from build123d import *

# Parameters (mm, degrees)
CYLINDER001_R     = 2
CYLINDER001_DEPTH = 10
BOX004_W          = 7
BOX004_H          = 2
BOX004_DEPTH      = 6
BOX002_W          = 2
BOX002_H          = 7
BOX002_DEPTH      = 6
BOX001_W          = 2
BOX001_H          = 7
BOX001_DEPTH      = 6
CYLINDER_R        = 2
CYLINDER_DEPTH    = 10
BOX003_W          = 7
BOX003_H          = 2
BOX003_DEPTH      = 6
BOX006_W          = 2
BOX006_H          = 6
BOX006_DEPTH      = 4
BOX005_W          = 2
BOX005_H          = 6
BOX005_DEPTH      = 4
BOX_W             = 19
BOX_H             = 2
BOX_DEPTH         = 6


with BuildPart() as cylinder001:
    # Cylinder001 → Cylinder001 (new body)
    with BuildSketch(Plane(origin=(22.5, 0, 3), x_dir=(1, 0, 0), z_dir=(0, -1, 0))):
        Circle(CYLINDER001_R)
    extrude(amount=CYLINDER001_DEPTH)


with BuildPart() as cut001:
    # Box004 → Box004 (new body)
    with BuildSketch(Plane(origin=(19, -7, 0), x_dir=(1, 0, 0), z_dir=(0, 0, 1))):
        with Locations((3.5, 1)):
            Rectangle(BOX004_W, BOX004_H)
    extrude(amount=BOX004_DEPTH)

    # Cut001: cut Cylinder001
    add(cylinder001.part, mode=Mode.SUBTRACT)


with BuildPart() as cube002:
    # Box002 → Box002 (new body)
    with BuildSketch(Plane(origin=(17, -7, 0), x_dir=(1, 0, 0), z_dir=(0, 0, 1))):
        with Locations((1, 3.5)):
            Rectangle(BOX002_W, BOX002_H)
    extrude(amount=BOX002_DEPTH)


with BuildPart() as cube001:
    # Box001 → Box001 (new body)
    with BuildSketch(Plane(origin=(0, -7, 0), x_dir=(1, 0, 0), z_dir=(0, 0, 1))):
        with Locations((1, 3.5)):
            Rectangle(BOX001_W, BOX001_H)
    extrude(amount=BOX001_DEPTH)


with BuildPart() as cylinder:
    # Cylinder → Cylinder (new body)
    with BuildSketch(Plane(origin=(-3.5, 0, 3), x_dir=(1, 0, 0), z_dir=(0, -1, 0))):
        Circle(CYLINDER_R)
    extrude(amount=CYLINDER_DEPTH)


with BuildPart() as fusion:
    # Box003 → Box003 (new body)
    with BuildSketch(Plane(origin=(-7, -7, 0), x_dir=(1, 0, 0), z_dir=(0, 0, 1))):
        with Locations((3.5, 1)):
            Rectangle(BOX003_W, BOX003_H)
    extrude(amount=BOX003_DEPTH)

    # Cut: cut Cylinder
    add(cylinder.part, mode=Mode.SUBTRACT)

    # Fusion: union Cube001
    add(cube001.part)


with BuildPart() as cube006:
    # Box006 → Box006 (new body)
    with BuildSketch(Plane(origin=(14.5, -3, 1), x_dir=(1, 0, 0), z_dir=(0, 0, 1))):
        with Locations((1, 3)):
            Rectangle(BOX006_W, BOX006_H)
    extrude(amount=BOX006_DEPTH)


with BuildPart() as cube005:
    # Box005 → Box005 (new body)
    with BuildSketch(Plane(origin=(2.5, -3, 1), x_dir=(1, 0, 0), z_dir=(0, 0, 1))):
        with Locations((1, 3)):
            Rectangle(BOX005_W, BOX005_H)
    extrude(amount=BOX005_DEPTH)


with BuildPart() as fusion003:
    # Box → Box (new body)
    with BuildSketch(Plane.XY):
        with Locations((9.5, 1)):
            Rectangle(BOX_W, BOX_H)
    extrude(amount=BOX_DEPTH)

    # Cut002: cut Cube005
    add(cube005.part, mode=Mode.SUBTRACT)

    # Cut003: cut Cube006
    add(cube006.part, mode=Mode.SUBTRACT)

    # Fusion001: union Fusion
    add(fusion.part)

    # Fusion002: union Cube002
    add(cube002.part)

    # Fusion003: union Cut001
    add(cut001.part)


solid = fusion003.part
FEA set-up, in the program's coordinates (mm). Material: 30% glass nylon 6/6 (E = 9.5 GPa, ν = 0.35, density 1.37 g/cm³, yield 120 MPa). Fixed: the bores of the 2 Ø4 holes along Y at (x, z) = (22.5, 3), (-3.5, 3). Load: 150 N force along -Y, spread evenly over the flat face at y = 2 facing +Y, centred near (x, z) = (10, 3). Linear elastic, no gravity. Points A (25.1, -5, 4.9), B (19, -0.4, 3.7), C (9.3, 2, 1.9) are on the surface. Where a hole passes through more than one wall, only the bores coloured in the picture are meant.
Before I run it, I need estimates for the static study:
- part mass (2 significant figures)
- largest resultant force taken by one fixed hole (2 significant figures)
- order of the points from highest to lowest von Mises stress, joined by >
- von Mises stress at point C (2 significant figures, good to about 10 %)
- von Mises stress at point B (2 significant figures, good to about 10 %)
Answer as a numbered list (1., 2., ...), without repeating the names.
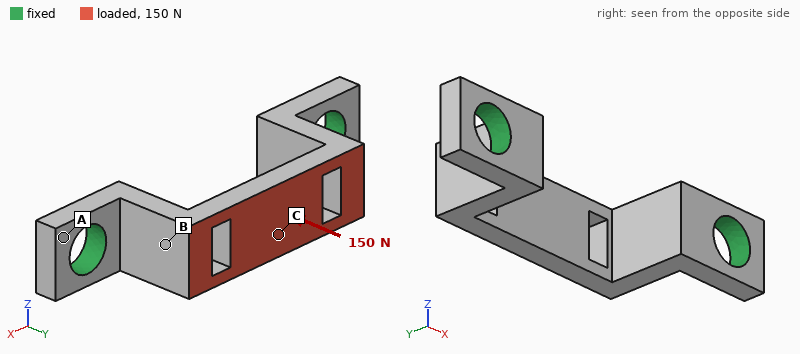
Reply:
1. 0.66 g
2. 84 N
3. C > B > A
4. 36 MPa
5. 16 MPa
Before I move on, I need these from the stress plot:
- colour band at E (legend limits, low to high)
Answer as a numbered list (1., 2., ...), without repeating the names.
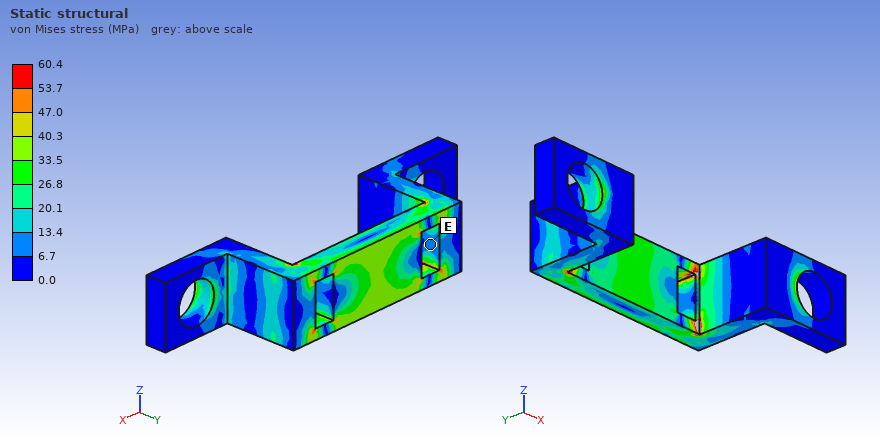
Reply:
1. 6.7 to 13.4 MPa
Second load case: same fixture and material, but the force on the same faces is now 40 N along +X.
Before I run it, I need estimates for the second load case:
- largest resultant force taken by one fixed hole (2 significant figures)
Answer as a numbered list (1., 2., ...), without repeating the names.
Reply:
1. 22 N
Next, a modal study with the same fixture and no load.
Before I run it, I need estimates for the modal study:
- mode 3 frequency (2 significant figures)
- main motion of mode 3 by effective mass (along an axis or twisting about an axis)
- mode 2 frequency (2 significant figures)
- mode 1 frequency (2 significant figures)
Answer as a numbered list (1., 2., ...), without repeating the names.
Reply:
1. 12 kHz
2. along Y
3. 7500 Hz
4. 7200 Hz
